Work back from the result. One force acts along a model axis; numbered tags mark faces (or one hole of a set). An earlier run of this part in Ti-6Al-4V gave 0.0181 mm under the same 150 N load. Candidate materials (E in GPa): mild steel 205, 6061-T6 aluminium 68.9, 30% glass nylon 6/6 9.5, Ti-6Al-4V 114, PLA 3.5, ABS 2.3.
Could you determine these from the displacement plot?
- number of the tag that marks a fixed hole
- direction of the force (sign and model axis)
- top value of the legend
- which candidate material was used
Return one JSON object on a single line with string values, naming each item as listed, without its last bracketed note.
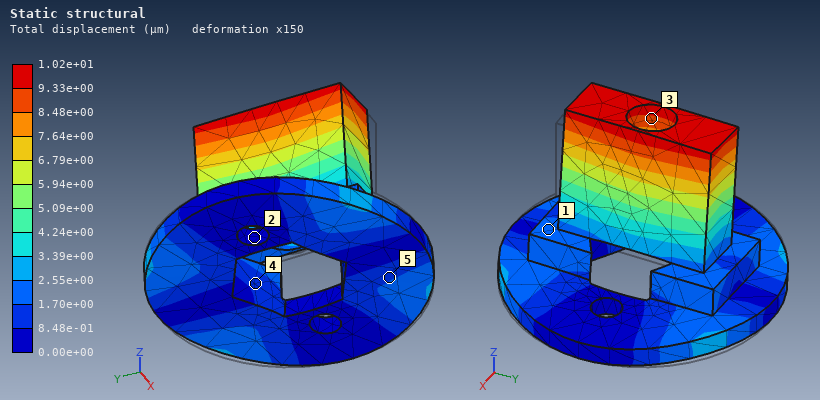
{"number of the tag that marks a fixed hole": "2", "direction of the force": "-X", "top value of the legend": "1.02e+01 µm", "which candidate material was used": "mild steel"}
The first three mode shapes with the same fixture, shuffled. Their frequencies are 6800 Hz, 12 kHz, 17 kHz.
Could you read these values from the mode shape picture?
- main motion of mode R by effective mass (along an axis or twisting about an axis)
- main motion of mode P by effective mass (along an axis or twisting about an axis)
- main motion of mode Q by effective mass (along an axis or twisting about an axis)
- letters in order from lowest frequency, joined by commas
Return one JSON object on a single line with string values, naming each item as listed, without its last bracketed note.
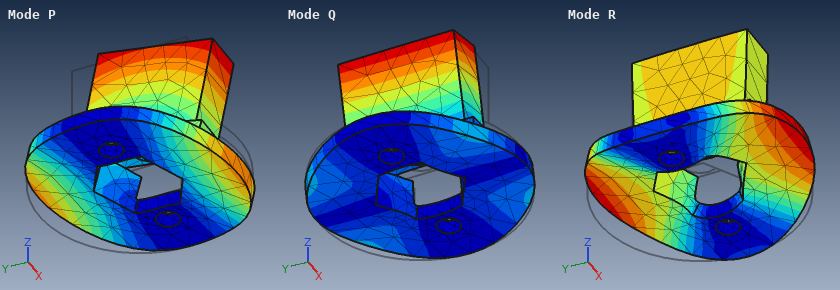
{"main motion of mode R by effective mass": "along Z", "main motion of mode P by effective mass": "along Y", "main motion of mode Q by effective mass": "along X", "letters in order from lowest frequency, joined by commas": "P, Q, R"}
